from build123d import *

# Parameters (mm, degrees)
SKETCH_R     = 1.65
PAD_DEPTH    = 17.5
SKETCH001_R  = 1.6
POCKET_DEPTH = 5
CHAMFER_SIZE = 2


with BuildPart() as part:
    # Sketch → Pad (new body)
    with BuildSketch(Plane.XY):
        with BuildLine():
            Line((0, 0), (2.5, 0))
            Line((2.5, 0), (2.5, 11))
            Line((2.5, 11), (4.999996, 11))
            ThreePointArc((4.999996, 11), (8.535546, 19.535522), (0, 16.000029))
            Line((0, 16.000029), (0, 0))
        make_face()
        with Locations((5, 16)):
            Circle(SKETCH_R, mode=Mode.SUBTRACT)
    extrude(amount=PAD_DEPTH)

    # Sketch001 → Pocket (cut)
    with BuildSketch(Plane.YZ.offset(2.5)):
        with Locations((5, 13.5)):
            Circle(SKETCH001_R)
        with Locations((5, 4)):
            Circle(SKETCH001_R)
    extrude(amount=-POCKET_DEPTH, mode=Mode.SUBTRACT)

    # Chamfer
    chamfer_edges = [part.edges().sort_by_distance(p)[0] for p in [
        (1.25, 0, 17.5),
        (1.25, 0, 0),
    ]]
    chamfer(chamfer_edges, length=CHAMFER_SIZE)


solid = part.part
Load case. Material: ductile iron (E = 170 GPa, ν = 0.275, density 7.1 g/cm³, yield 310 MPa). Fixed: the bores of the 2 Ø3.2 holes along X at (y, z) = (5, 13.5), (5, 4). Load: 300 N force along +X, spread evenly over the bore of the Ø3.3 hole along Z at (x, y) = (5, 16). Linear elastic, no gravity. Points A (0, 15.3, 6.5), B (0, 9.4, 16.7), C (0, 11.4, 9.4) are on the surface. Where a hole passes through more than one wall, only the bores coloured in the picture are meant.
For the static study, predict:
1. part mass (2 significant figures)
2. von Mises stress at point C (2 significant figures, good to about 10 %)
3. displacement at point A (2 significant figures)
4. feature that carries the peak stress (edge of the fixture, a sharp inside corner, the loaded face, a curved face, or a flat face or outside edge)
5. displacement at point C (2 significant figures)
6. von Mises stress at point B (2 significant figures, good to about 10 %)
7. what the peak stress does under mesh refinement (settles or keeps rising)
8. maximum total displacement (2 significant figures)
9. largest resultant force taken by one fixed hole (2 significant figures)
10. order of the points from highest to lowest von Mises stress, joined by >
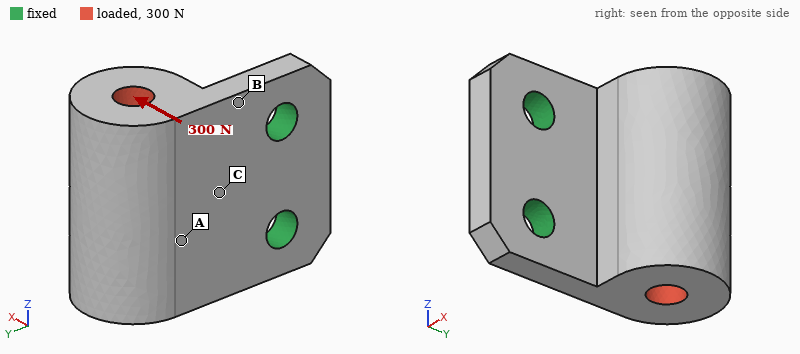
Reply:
12 g
61 MPa
24 µm
edge of the fixture
11 µm
100 MPa
keeps rising
46 µm
150 N
B > C > A
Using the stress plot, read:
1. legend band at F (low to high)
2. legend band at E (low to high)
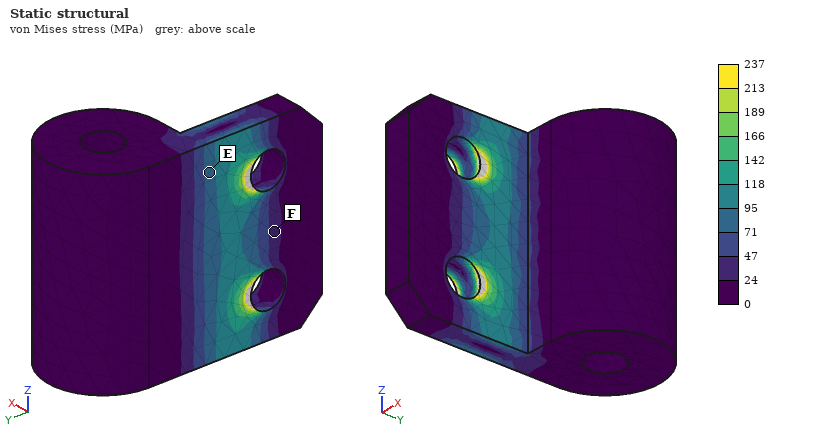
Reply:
24 to 47 MPa
71 to 95 MPa
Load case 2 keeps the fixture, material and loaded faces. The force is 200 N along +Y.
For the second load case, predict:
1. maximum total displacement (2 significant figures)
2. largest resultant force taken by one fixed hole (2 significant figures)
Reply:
16 µm
100 N
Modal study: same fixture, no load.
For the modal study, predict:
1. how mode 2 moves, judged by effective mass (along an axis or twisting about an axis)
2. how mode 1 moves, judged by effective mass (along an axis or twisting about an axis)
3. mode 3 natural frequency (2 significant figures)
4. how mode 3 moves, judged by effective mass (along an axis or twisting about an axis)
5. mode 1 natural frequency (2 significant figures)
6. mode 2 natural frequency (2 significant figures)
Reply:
along Z
along X
23 kHz
along Z
4700 Hz
13 kHz
